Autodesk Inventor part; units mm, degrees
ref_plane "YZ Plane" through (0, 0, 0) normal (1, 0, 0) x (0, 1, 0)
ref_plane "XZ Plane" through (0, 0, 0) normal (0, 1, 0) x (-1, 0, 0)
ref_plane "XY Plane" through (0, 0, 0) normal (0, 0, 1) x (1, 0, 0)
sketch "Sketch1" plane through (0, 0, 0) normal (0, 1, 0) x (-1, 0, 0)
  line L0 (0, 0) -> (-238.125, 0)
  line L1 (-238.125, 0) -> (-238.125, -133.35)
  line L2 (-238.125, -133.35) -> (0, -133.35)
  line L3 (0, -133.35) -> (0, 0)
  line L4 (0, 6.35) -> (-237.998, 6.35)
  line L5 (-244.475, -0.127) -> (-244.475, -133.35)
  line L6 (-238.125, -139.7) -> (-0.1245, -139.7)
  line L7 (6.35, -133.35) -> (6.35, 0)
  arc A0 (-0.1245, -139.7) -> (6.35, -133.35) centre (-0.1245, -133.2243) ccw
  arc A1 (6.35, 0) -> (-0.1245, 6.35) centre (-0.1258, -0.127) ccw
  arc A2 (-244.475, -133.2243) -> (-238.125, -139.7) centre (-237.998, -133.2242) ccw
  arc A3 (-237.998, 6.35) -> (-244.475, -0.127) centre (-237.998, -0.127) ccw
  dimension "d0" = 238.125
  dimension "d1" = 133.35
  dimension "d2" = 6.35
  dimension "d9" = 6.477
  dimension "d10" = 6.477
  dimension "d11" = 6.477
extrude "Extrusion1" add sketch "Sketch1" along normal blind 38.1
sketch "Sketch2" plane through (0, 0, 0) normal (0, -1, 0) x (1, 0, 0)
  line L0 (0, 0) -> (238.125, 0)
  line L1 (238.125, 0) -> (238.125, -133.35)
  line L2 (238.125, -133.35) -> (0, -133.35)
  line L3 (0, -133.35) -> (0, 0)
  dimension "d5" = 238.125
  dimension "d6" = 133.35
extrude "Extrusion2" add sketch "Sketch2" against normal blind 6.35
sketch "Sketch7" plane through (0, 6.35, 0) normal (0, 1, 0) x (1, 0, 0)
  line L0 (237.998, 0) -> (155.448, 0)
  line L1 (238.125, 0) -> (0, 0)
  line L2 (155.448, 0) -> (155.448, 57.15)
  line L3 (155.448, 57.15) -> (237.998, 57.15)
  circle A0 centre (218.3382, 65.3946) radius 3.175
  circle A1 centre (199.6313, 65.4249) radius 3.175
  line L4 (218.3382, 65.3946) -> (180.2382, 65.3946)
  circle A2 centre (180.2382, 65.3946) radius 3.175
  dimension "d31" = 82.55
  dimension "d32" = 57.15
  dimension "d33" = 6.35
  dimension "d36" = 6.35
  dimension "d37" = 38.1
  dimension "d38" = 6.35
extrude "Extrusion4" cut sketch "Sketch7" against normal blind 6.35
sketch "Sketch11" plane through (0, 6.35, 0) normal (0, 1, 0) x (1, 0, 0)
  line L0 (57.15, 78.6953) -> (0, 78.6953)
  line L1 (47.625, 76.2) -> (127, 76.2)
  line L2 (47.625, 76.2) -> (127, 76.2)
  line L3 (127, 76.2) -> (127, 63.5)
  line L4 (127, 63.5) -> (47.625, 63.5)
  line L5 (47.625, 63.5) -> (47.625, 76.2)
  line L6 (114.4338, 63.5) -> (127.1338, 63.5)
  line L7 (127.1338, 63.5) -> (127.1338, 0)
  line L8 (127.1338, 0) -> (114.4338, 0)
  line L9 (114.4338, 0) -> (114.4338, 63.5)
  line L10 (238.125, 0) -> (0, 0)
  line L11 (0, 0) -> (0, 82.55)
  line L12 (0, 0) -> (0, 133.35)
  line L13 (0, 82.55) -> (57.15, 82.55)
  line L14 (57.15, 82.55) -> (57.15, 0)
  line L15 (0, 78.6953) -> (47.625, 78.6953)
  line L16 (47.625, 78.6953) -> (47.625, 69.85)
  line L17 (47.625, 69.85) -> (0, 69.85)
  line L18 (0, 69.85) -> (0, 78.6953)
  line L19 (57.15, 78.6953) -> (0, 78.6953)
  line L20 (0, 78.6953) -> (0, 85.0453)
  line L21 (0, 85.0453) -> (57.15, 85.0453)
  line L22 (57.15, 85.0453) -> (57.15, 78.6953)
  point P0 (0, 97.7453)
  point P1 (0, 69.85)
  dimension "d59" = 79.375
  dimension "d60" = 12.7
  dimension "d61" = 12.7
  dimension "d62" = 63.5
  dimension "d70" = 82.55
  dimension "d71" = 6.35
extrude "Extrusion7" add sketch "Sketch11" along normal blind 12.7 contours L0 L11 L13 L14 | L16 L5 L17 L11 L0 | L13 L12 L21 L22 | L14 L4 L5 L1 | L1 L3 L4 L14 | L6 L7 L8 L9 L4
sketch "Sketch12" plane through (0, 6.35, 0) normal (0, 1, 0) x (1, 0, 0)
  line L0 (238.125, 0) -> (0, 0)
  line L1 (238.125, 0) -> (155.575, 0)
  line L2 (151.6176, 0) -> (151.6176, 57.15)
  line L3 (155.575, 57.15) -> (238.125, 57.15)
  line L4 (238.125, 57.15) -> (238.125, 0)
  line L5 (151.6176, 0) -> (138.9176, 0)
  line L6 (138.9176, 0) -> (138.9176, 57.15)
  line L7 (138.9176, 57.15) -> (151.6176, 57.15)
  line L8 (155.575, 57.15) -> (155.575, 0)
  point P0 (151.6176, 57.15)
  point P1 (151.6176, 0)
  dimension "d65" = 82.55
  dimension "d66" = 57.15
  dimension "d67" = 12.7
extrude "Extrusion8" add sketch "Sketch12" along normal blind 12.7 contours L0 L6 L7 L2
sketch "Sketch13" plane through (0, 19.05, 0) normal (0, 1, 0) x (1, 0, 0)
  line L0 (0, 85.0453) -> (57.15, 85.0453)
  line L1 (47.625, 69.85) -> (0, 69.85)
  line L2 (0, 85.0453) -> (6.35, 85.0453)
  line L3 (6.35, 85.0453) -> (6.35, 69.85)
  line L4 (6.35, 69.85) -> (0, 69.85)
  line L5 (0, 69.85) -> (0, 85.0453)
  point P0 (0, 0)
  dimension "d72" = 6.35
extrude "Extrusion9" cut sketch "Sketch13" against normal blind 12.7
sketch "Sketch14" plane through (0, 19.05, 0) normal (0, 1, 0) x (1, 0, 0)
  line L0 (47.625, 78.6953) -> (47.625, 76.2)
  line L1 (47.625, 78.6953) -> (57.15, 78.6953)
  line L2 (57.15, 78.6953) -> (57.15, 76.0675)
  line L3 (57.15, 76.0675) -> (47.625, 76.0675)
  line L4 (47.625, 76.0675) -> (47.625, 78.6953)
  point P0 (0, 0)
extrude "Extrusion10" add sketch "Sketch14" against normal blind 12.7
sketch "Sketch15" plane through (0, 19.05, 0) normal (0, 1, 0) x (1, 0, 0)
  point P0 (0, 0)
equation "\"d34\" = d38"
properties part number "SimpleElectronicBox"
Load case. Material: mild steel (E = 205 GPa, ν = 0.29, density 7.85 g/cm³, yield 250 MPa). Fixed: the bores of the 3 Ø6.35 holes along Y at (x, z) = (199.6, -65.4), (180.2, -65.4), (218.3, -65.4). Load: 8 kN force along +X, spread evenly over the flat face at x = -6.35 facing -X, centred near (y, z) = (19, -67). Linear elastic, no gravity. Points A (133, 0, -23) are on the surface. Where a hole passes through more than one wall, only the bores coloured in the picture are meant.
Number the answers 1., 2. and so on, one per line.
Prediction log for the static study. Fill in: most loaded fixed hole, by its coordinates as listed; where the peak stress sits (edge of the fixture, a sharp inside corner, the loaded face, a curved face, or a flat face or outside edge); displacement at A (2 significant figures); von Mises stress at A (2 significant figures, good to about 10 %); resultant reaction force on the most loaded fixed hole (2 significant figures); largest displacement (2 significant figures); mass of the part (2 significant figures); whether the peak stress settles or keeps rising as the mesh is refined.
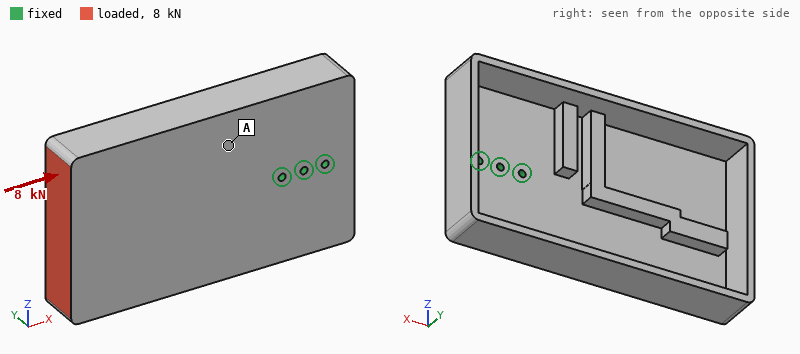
1. (180.2, -65.4)
2. edge of the fixture
3. 0.12 mm
4. 12 MPa
5. 4.7 kN
6. 0.50 mm
7. 3.4 kg
8. keeps rising
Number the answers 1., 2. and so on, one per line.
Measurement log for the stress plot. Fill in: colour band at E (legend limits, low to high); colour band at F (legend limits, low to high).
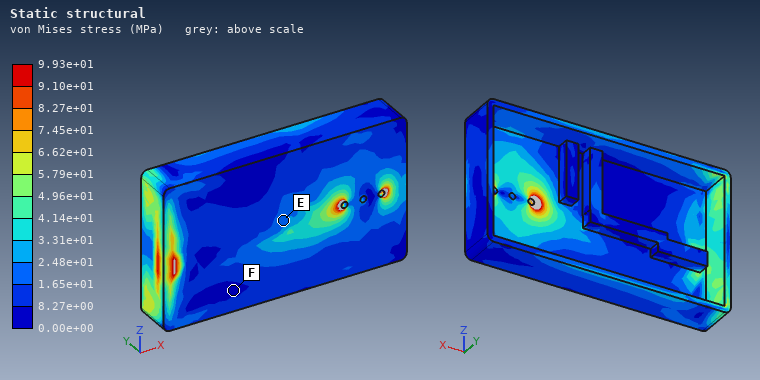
1. 1.65e+01 to 2.48e+01 MPa
2. 0.00e+00 to 8.27e+00 MPa
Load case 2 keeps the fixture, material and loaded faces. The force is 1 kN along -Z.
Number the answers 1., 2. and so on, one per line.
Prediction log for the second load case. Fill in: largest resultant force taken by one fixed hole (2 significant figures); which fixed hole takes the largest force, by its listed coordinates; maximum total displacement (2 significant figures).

1. 5.3 kN
2. (180.2, -65.4)
3. 0.13 mm
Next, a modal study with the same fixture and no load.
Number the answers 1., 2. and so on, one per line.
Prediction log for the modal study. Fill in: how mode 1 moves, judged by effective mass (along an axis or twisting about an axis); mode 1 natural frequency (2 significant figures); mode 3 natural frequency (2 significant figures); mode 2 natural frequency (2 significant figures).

1. along Y
2. 190 Hz
3. 730 Hz
4. 290 Hz
